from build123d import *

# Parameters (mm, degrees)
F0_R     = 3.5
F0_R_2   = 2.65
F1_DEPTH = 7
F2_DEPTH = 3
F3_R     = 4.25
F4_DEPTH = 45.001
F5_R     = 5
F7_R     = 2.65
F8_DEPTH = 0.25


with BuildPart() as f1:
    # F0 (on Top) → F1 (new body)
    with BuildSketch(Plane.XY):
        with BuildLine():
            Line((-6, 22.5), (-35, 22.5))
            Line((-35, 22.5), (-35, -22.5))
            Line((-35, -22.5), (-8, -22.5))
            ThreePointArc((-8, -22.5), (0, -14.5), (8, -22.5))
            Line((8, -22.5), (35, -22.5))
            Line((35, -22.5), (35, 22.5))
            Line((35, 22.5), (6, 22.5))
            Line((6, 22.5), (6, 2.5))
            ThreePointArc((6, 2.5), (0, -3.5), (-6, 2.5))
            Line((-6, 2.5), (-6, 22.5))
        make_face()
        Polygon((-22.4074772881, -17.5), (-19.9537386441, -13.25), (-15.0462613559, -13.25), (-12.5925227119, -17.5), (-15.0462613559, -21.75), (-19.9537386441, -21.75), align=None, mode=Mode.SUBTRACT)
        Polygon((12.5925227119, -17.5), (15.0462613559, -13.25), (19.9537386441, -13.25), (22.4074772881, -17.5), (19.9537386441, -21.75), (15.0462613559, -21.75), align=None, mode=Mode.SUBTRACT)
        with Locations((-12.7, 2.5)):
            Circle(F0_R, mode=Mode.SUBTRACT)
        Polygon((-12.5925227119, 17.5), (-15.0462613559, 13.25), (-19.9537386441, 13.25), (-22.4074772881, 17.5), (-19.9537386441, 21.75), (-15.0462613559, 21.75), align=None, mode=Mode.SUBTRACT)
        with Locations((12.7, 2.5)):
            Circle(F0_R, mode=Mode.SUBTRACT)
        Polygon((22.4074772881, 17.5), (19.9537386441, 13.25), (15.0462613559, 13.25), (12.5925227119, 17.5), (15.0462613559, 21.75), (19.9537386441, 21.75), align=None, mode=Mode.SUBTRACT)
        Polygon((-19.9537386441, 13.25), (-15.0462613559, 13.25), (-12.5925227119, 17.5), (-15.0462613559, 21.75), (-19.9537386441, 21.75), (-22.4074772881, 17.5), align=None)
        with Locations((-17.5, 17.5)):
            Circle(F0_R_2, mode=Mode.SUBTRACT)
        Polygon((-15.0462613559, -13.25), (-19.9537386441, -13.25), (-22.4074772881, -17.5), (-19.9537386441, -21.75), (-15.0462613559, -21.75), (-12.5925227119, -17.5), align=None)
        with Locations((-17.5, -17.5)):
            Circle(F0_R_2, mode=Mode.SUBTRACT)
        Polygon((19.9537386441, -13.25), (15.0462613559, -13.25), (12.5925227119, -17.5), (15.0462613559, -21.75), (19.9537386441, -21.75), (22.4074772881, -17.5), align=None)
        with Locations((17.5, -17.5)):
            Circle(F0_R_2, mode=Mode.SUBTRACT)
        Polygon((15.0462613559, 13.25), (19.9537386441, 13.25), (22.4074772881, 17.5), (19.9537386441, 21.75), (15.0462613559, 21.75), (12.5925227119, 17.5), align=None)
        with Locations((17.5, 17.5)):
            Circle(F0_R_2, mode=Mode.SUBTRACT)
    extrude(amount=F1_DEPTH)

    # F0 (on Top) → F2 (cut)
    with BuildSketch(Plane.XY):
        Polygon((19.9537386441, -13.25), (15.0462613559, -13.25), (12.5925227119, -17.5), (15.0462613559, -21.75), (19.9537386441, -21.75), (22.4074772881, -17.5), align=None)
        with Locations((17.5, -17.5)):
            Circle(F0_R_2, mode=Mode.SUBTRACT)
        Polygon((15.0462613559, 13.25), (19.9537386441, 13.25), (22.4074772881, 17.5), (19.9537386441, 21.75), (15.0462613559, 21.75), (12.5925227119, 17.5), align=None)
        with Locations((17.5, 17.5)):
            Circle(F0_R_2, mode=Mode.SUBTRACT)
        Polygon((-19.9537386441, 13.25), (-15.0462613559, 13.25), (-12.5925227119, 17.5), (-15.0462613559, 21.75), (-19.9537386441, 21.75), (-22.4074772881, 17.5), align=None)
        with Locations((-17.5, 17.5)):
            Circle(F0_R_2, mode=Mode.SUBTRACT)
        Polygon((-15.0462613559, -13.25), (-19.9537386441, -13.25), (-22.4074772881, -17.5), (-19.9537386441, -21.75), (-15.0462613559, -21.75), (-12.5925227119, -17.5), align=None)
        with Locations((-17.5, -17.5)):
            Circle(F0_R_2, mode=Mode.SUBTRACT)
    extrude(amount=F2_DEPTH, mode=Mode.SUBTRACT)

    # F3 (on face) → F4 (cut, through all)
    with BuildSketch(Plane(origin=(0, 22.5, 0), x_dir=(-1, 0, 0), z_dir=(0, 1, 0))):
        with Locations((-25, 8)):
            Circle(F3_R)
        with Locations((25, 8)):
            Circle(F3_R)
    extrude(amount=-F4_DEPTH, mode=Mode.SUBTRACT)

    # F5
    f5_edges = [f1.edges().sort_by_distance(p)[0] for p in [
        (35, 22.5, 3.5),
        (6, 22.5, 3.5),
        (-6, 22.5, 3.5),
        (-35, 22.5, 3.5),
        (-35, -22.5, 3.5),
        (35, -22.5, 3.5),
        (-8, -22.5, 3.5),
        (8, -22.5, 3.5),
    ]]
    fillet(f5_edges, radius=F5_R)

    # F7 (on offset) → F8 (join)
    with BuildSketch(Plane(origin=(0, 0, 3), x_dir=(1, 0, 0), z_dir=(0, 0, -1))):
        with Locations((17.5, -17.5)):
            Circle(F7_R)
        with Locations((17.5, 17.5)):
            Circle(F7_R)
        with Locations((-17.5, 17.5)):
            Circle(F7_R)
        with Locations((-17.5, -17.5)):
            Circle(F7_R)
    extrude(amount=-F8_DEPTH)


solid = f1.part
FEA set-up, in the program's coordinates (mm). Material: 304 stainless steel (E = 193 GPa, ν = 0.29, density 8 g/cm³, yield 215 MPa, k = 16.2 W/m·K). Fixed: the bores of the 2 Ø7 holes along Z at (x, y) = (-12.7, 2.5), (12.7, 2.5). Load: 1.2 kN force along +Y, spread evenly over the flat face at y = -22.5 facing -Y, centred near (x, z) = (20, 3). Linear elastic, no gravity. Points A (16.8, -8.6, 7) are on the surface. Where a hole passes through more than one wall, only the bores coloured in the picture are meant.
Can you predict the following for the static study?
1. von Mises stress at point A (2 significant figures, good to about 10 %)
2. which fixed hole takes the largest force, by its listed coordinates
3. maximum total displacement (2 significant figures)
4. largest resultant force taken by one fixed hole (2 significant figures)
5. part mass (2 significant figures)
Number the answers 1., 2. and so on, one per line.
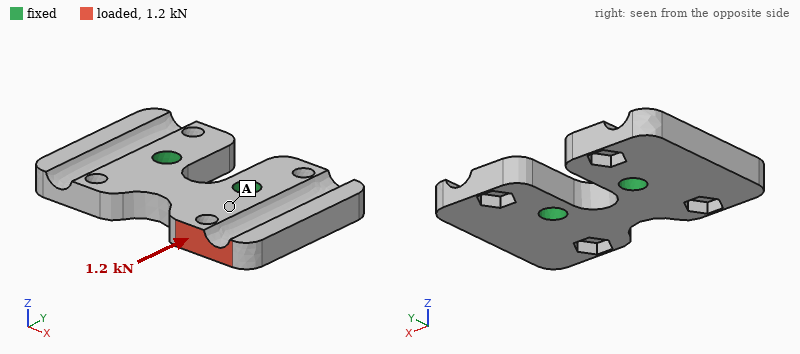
1. 9.9 MPa
2. (12.7, 2.5)
3. 6.9 µm
4. 1.3 kN
5. 120 g
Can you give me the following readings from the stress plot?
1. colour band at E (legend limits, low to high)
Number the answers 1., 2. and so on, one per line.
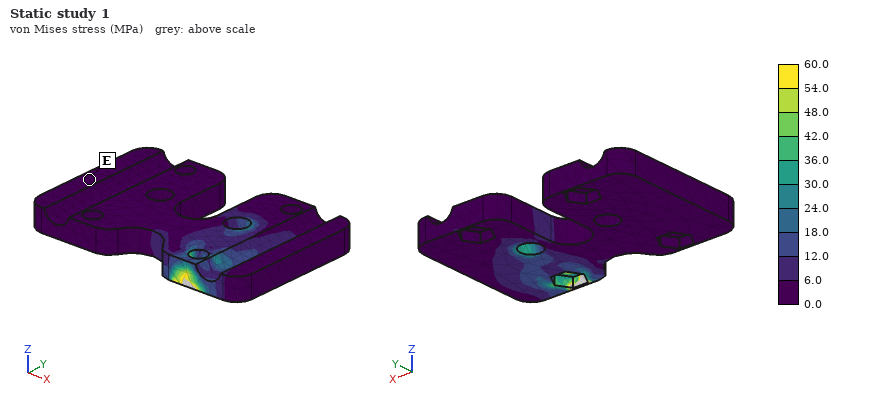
1. 0.0 to 6.0 MPa
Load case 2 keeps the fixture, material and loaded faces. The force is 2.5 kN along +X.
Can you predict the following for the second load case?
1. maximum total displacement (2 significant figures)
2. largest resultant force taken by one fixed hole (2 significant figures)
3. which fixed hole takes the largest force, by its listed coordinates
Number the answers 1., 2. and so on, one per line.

1. 17 µm
2. 2.2 kN
3. (-12.7, 2.5)
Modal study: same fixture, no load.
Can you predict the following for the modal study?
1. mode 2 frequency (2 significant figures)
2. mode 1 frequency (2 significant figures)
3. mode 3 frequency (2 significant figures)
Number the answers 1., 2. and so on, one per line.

1. 7400 Hz
2. 7300 Hz
3. 8400 Hz
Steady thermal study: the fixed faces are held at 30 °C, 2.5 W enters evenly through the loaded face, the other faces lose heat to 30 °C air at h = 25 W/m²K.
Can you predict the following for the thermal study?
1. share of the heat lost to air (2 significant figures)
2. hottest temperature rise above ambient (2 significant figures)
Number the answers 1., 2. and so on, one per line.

1. 26 %
2. 31 K
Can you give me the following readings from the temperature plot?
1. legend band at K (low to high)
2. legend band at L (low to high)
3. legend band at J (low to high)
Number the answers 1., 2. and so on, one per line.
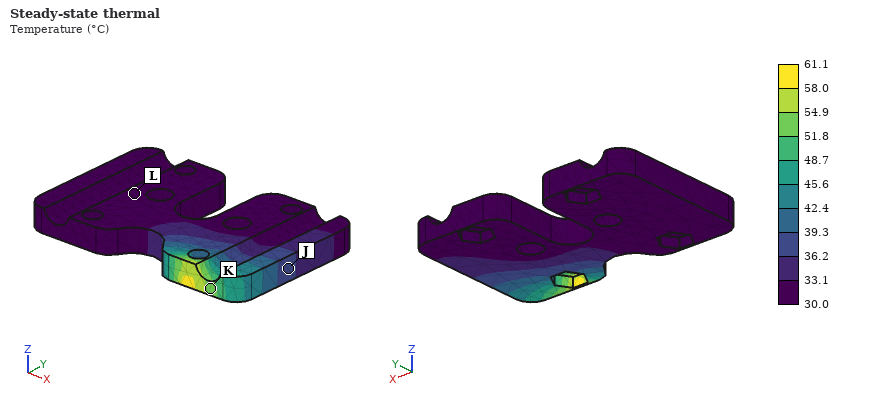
1. 51.8 to 54.9 °C
2. 30.0 to 33.1 °C
3. 36.2 to 39.3 °C
